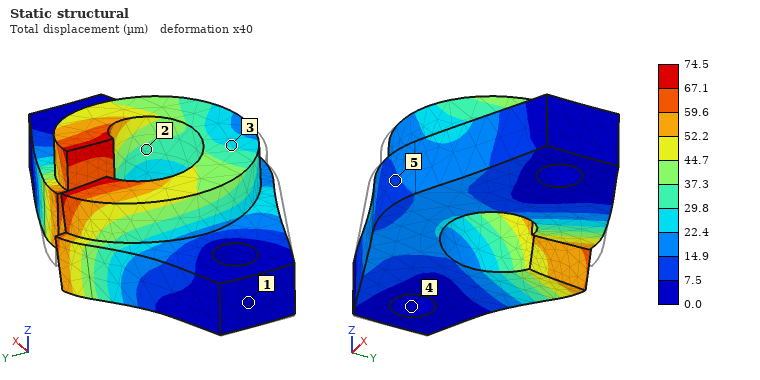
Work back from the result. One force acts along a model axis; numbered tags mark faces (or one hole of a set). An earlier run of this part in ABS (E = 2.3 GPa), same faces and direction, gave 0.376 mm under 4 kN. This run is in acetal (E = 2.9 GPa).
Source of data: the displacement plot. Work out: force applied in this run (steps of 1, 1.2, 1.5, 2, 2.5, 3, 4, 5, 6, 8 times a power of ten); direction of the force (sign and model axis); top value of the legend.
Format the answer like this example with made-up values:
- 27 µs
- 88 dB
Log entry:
- 1 kN
- +X
- 74.5 µm
